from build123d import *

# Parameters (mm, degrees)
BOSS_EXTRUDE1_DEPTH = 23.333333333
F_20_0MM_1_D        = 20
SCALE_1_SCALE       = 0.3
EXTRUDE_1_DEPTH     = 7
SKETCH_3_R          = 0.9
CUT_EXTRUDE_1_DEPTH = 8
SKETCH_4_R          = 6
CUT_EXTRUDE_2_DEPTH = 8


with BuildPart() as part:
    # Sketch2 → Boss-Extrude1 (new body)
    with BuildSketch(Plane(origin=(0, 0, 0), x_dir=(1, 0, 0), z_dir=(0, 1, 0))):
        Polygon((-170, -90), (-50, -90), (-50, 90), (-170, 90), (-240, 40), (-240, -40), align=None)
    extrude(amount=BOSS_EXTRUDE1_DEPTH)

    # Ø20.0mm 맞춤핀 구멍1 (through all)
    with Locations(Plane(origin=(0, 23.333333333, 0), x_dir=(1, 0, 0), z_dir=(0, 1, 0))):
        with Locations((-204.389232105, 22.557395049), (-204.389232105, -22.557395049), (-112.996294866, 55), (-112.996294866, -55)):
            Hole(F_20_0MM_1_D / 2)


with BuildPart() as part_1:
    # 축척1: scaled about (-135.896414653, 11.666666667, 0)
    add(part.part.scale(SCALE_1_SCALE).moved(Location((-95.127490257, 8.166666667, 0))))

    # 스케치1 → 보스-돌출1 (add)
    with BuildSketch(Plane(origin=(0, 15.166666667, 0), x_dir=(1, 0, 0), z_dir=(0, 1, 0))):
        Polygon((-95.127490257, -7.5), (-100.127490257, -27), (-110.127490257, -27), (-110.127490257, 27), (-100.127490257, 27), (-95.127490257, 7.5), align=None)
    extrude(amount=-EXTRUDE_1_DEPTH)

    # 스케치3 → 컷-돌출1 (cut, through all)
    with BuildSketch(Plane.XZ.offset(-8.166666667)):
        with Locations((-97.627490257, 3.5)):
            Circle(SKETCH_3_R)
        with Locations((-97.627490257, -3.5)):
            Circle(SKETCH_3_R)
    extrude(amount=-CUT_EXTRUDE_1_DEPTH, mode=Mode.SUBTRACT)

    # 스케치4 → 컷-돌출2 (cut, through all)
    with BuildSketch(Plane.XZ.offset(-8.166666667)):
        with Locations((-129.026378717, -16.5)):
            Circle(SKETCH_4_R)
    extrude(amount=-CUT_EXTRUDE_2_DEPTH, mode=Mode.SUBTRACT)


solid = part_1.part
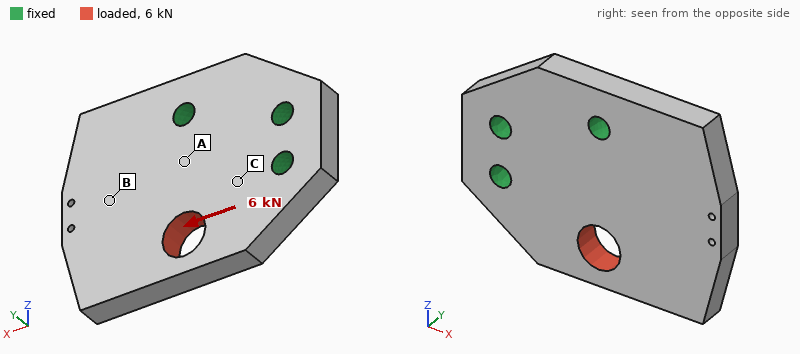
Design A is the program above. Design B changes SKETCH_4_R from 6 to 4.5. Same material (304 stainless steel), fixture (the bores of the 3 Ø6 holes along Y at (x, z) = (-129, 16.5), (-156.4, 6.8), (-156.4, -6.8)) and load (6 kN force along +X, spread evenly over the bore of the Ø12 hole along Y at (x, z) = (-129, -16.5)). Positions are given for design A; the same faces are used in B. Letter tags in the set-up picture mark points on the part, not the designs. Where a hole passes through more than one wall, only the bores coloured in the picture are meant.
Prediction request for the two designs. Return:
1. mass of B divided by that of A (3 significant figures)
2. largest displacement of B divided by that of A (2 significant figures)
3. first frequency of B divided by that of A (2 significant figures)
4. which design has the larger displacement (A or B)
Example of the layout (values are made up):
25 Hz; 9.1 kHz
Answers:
1.02; 0.90; 1.0; A
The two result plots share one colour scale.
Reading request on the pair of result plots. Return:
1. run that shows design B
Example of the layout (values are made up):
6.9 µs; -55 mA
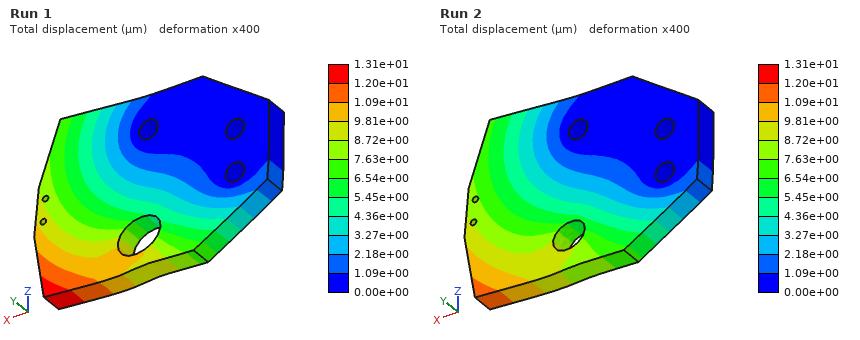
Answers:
Run 2
